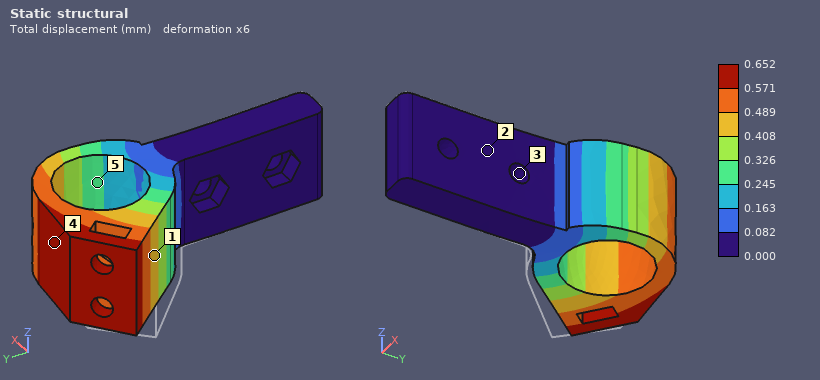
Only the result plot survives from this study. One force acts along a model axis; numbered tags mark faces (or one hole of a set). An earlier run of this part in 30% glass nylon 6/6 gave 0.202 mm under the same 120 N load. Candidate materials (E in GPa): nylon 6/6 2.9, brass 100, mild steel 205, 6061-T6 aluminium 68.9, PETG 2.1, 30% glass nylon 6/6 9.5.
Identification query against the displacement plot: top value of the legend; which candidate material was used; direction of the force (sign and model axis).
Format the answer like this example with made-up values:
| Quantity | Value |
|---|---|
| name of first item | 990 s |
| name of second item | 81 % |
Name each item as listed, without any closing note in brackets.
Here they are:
| Quantity | Value |
|---|---|
| top value of the legend | 0.652 mm |
| which candidate material was used | nylon 6/6 |
| direction of the force | +X |
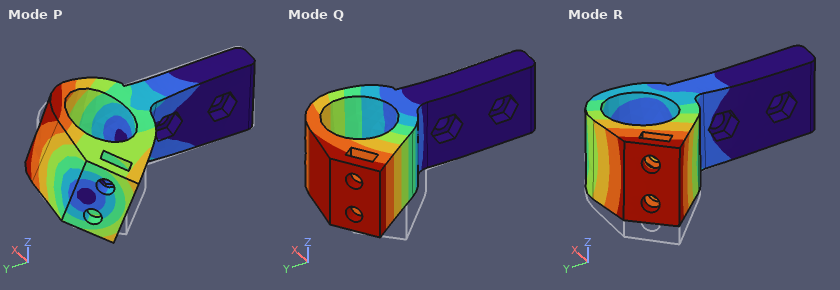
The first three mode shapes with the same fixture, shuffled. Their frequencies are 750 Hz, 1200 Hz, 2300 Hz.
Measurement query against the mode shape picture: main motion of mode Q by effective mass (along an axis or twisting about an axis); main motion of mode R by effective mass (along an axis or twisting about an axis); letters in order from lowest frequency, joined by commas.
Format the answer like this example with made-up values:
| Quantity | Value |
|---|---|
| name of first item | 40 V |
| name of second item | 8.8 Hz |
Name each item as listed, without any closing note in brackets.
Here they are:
| Quantity | Value |
|---|---|
| main motion of mode Q by effective mass | along X |
| main motion of mode R by effective mass | along Z |
| letters in order from lowest frequency, joined by commas | Q, R, P |
